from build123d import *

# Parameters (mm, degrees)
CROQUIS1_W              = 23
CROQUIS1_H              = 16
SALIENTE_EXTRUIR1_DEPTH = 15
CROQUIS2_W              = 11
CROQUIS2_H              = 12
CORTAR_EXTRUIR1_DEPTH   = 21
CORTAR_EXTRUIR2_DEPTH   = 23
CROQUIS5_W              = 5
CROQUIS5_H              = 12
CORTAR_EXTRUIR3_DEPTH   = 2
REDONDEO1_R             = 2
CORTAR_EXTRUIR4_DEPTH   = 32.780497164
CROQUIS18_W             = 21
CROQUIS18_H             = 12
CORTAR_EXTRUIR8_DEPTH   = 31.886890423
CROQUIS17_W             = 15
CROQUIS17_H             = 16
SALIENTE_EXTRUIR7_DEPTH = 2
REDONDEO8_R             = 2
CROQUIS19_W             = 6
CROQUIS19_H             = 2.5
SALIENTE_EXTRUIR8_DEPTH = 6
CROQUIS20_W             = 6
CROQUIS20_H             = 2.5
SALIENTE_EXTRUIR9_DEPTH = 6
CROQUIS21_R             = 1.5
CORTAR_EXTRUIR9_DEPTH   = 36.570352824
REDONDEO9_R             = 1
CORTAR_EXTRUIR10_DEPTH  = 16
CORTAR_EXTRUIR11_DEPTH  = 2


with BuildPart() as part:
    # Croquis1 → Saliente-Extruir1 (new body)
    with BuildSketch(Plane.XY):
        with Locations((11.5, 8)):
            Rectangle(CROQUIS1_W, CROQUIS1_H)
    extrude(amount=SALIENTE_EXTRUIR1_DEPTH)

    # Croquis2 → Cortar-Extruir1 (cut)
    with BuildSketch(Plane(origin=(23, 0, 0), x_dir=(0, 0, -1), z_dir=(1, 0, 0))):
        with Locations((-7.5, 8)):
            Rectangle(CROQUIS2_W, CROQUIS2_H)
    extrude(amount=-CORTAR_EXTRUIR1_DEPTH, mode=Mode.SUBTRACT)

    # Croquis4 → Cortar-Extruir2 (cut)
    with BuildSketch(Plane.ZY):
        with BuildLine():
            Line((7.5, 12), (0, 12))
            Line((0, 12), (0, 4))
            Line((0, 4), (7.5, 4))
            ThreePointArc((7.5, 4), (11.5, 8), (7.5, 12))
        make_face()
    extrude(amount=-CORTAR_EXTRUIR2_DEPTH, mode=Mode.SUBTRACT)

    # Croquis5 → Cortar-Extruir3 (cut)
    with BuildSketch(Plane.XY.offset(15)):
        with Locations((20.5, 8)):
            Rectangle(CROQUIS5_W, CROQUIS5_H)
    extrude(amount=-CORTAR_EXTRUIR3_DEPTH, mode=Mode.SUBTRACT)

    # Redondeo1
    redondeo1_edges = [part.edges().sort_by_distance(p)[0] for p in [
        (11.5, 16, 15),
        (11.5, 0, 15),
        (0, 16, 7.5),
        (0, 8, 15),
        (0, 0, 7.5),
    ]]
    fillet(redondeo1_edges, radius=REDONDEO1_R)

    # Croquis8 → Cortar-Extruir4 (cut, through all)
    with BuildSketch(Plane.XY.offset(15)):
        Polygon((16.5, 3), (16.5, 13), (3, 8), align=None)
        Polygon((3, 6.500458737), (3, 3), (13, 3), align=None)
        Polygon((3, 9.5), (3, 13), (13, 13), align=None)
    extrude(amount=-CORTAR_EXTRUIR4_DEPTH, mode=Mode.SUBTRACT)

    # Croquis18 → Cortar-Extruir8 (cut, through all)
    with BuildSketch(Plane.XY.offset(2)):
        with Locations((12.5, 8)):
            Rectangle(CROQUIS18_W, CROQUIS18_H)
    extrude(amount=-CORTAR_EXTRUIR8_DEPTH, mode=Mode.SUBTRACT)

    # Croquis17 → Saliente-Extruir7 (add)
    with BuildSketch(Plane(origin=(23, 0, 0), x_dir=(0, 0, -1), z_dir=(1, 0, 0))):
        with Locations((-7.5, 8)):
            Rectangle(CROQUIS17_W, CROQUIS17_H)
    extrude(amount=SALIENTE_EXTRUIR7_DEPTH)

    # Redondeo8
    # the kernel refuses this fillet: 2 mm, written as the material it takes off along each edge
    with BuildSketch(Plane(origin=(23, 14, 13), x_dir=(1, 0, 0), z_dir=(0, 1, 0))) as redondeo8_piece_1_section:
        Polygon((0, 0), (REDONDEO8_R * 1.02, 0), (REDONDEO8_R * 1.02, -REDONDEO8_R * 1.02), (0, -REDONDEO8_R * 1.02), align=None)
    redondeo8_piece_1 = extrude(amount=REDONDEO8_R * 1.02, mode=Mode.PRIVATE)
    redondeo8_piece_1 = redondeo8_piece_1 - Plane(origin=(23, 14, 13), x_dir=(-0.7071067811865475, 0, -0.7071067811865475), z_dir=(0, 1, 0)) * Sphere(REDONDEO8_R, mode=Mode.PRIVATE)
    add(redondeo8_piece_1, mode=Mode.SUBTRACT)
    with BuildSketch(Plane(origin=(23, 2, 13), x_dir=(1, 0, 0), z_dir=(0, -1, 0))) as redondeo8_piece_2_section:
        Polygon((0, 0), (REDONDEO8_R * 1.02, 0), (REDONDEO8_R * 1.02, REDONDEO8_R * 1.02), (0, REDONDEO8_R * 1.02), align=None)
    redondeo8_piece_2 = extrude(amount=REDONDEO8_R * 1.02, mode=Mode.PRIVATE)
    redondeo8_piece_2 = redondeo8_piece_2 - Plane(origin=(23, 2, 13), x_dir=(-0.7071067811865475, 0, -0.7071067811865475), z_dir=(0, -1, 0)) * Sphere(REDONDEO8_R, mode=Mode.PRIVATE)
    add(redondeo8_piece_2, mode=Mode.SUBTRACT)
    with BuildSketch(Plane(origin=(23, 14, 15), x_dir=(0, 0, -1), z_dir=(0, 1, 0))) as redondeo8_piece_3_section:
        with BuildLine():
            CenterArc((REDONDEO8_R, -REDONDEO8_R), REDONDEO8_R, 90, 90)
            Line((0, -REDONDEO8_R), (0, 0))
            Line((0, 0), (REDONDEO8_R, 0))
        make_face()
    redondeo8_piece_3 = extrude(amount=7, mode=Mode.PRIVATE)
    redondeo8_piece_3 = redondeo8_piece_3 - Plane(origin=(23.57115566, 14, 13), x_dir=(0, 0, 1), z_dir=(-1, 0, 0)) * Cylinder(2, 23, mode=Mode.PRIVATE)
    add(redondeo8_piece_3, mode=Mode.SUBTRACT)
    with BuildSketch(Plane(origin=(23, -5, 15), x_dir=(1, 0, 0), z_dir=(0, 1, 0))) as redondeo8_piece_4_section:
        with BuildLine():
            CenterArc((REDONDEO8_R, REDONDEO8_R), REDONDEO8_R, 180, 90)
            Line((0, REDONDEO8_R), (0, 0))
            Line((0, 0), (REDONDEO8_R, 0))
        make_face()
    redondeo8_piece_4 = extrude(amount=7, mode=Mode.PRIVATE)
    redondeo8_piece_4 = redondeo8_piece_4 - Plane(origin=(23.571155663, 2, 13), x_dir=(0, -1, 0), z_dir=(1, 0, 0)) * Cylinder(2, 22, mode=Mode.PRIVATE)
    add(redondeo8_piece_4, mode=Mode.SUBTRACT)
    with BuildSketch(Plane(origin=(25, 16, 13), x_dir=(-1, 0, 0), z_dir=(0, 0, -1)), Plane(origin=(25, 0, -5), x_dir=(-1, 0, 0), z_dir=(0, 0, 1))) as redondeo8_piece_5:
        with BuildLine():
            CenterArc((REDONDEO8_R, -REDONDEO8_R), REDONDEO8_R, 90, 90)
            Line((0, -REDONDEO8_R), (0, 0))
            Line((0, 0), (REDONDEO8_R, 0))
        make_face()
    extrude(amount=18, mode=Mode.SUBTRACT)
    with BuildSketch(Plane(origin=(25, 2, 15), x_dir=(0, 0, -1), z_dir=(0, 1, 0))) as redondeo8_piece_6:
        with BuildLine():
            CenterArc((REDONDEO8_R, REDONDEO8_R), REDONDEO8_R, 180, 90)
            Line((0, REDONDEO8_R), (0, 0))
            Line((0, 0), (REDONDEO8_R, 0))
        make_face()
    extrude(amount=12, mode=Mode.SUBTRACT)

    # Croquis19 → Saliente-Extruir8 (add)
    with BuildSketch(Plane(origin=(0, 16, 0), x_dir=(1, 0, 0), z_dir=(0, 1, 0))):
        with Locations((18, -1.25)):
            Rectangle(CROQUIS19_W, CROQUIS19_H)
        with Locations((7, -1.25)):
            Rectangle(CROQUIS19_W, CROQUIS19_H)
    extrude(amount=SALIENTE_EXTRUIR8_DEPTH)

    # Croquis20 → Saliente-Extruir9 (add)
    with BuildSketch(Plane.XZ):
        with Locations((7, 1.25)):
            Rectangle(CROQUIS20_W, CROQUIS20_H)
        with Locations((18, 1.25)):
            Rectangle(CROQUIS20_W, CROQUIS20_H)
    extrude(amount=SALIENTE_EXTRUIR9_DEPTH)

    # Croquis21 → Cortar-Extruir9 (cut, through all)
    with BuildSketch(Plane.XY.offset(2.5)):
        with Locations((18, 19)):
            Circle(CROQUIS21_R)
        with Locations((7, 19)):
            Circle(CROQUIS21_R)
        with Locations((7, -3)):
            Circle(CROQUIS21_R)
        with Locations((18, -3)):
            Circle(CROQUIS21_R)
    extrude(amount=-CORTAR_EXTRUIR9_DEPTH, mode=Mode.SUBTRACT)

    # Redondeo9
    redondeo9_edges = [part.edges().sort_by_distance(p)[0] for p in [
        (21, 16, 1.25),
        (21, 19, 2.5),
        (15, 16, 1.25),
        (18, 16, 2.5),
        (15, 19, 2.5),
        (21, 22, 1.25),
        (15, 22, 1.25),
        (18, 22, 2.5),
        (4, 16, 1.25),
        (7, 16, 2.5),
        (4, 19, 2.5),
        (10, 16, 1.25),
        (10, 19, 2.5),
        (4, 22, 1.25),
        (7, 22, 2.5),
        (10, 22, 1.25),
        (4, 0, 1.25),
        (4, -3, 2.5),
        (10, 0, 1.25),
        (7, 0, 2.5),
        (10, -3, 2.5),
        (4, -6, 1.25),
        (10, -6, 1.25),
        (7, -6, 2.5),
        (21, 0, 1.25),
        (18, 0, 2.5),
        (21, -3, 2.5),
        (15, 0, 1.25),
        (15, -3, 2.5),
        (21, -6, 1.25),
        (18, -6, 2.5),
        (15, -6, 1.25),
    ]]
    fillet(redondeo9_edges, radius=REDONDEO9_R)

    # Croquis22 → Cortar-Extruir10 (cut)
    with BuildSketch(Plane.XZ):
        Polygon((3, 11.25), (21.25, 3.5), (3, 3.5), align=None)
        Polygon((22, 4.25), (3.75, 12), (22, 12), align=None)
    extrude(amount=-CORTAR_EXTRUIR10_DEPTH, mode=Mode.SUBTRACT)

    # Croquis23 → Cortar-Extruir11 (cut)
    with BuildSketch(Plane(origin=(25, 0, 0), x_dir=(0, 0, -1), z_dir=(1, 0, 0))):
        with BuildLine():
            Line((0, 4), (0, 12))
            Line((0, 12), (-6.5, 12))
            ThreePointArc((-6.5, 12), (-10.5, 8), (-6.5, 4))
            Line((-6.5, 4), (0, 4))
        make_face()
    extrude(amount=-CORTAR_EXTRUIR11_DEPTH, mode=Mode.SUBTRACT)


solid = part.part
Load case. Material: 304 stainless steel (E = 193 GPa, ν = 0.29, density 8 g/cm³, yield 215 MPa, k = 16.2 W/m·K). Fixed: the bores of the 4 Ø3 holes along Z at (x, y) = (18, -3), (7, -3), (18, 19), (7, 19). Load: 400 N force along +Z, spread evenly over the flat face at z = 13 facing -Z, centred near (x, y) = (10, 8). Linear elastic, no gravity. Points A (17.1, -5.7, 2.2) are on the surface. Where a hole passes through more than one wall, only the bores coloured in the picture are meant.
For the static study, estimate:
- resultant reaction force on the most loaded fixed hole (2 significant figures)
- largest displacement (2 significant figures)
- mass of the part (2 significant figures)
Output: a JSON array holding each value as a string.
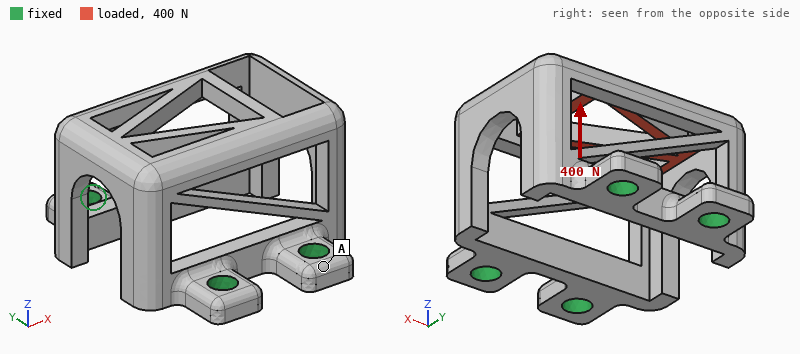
["140 N", "26 µm", "13 g"]
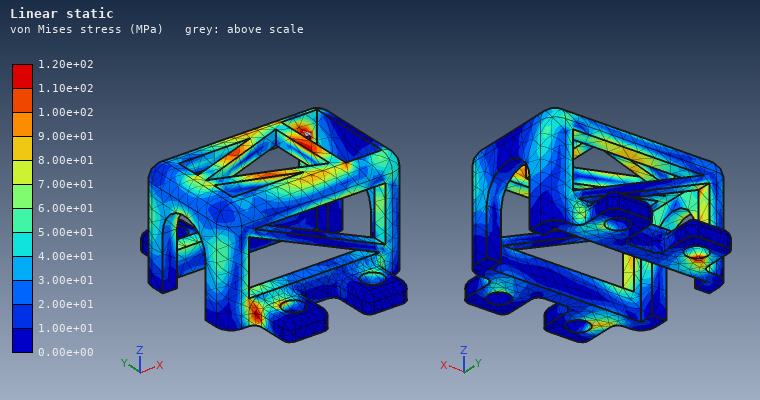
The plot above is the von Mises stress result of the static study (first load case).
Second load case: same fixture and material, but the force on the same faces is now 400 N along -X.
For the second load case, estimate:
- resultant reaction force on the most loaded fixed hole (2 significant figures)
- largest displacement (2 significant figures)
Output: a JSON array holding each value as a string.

["180 N", "28 µm"]
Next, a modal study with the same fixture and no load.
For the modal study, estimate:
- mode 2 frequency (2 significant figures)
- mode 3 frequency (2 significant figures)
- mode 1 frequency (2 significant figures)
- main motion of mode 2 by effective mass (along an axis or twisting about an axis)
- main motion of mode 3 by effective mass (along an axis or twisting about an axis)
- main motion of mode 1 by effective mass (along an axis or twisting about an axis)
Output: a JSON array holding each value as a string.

["9200 Hz", "11 kHz", "8100 Hz", "along Y", "along Z", "along X"]
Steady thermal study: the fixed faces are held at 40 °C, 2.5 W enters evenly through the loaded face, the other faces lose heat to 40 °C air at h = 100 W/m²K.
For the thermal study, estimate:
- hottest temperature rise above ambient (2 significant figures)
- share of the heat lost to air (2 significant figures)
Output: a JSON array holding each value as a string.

["33 K", "88 %"]
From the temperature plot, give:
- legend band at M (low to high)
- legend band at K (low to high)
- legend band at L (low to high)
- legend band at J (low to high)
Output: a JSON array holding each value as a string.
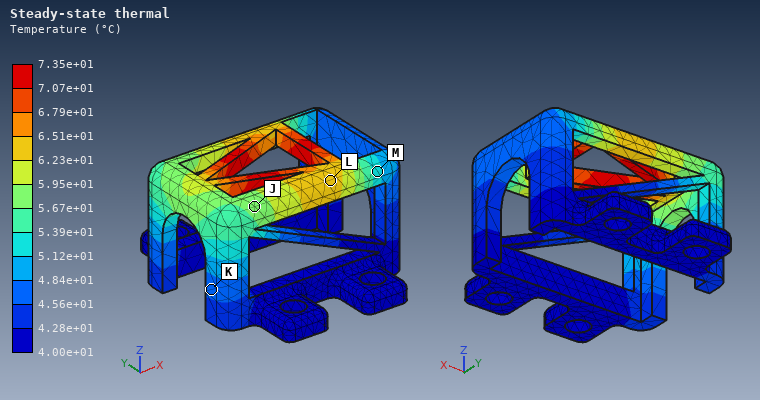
["5.12e+01 to 5.39e+01 °C", "4.56e+01 to 4.84e+01 °C", "6.23e+01 to 6.51e+01 °C", "5.67e+01 to 5.95e+01 °C"]
